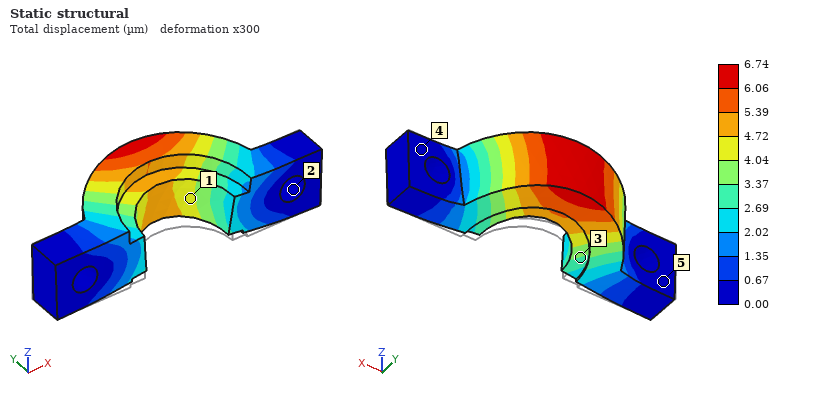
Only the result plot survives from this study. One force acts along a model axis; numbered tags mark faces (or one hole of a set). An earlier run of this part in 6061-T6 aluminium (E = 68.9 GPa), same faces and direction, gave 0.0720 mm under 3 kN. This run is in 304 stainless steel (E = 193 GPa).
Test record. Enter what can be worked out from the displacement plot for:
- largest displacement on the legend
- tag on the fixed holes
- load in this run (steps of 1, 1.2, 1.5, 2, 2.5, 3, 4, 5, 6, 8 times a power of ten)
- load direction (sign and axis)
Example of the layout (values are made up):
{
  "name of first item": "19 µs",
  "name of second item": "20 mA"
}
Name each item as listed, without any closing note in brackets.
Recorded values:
{
  "largest displacement on the legend": "6.74 µm",
  "tag on the fixed holes": "2",
  "load in this run": "800 N",
  "load direction": "+Z"
}
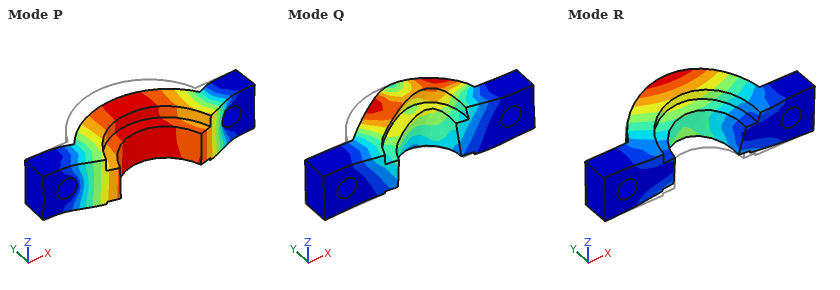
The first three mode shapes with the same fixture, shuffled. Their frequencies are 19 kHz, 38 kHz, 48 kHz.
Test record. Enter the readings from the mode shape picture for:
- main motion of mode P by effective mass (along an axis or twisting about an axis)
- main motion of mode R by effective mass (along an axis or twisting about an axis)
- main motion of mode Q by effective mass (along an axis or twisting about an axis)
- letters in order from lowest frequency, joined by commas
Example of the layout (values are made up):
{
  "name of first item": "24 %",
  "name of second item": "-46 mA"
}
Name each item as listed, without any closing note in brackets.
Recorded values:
{
  "main motion of mode P by effective mass": "along Y",
  "main motion of mode R by effective mass": "along Z",
  "main motion of mode Q by effective mass": "along X",
  "letters in order from lowest frequency, joined by commas": "R, P, Q"
}
